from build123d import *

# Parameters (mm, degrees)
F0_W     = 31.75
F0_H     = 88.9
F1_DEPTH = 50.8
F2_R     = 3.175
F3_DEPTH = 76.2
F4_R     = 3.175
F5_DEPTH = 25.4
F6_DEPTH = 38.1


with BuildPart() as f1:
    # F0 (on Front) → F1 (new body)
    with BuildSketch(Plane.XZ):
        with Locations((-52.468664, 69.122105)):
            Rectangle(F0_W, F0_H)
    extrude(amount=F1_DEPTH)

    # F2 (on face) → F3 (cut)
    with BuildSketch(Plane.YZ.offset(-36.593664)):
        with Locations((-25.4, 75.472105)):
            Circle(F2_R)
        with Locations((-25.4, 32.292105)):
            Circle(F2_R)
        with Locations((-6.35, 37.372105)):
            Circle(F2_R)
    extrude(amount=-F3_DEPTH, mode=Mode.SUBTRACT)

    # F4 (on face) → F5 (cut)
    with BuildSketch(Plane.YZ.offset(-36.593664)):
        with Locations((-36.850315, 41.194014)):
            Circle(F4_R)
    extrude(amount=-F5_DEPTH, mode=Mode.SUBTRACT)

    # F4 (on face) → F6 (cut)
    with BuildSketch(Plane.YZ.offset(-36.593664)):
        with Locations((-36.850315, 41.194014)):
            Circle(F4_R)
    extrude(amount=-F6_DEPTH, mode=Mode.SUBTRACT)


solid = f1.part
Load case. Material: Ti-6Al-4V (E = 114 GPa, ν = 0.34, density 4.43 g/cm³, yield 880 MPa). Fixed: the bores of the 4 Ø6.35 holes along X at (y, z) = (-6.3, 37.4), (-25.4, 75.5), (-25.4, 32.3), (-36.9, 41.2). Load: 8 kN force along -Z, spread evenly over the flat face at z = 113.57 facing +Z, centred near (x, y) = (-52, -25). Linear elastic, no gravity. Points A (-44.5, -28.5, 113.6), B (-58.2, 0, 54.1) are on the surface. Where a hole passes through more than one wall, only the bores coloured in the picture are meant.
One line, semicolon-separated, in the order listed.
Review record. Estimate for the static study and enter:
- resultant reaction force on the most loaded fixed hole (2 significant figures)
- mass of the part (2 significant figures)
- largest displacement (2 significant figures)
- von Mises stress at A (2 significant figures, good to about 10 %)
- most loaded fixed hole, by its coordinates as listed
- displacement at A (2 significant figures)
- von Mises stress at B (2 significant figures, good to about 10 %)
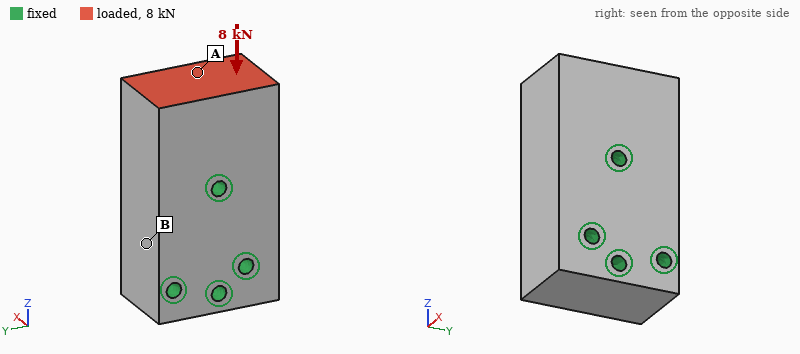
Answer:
5.4 kN; 620 g; 2.3 µm; 5.5 MPa; (-25.4, 75.5); 2.1 µm; 2.5 MPa
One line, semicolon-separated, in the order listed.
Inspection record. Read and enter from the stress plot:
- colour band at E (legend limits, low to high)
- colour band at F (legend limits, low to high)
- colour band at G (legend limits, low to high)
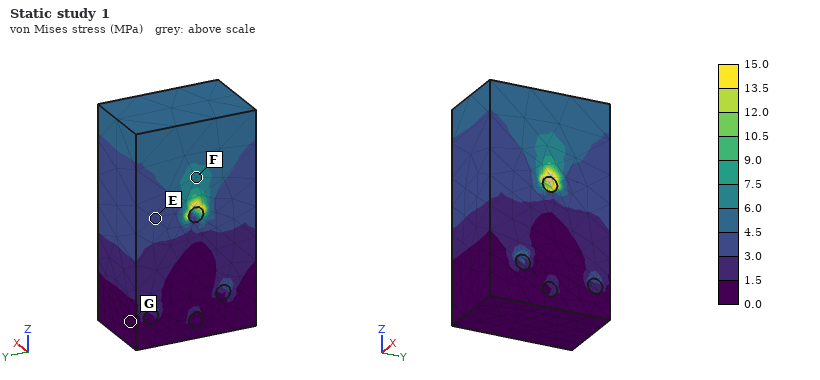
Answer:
3.0 to 4.5 MPa; 6.0 to 7.5 MPa; 0.0 to 1.5 MPa
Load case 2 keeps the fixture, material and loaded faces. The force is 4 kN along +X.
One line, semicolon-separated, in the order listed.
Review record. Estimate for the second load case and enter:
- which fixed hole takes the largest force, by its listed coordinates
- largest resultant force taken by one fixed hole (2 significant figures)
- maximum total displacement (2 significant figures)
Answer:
(-25.4, 75.5); 5.1 kN; 11 µm
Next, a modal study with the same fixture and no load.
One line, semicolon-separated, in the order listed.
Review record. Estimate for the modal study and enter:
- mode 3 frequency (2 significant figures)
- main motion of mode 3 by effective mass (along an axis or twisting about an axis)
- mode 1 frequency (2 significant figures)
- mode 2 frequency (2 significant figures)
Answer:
14 kHz; twisting about Z; 10 kHz; 10 kHz
